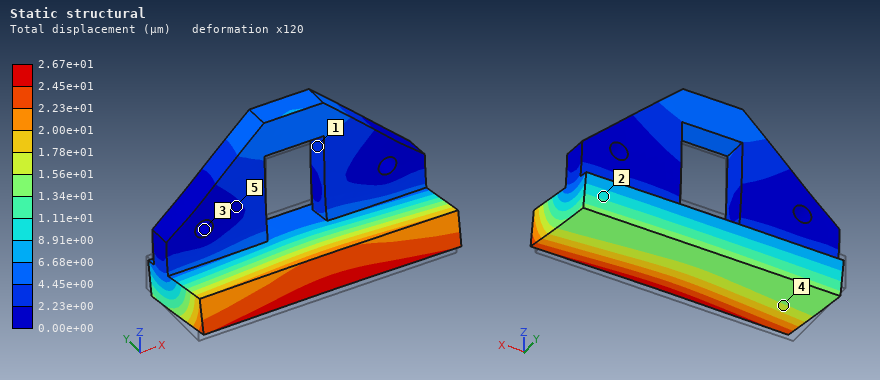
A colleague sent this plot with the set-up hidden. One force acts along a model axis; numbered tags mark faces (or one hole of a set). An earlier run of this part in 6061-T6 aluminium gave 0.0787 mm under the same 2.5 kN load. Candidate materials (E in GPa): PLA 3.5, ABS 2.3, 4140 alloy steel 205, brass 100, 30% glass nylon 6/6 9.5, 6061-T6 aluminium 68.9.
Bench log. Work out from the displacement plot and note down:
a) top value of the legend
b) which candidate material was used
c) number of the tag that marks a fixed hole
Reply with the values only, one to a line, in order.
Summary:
2.67e+01 µm
4140 alloy steel
3
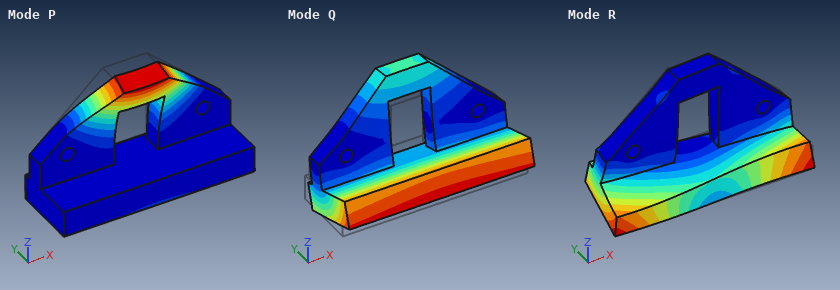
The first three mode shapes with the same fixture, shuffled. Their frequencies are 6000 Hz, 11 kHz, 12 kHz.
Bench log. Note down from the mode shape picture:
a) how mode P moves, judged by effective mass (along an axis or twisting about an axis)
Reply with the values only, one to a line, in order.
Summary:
along Y
